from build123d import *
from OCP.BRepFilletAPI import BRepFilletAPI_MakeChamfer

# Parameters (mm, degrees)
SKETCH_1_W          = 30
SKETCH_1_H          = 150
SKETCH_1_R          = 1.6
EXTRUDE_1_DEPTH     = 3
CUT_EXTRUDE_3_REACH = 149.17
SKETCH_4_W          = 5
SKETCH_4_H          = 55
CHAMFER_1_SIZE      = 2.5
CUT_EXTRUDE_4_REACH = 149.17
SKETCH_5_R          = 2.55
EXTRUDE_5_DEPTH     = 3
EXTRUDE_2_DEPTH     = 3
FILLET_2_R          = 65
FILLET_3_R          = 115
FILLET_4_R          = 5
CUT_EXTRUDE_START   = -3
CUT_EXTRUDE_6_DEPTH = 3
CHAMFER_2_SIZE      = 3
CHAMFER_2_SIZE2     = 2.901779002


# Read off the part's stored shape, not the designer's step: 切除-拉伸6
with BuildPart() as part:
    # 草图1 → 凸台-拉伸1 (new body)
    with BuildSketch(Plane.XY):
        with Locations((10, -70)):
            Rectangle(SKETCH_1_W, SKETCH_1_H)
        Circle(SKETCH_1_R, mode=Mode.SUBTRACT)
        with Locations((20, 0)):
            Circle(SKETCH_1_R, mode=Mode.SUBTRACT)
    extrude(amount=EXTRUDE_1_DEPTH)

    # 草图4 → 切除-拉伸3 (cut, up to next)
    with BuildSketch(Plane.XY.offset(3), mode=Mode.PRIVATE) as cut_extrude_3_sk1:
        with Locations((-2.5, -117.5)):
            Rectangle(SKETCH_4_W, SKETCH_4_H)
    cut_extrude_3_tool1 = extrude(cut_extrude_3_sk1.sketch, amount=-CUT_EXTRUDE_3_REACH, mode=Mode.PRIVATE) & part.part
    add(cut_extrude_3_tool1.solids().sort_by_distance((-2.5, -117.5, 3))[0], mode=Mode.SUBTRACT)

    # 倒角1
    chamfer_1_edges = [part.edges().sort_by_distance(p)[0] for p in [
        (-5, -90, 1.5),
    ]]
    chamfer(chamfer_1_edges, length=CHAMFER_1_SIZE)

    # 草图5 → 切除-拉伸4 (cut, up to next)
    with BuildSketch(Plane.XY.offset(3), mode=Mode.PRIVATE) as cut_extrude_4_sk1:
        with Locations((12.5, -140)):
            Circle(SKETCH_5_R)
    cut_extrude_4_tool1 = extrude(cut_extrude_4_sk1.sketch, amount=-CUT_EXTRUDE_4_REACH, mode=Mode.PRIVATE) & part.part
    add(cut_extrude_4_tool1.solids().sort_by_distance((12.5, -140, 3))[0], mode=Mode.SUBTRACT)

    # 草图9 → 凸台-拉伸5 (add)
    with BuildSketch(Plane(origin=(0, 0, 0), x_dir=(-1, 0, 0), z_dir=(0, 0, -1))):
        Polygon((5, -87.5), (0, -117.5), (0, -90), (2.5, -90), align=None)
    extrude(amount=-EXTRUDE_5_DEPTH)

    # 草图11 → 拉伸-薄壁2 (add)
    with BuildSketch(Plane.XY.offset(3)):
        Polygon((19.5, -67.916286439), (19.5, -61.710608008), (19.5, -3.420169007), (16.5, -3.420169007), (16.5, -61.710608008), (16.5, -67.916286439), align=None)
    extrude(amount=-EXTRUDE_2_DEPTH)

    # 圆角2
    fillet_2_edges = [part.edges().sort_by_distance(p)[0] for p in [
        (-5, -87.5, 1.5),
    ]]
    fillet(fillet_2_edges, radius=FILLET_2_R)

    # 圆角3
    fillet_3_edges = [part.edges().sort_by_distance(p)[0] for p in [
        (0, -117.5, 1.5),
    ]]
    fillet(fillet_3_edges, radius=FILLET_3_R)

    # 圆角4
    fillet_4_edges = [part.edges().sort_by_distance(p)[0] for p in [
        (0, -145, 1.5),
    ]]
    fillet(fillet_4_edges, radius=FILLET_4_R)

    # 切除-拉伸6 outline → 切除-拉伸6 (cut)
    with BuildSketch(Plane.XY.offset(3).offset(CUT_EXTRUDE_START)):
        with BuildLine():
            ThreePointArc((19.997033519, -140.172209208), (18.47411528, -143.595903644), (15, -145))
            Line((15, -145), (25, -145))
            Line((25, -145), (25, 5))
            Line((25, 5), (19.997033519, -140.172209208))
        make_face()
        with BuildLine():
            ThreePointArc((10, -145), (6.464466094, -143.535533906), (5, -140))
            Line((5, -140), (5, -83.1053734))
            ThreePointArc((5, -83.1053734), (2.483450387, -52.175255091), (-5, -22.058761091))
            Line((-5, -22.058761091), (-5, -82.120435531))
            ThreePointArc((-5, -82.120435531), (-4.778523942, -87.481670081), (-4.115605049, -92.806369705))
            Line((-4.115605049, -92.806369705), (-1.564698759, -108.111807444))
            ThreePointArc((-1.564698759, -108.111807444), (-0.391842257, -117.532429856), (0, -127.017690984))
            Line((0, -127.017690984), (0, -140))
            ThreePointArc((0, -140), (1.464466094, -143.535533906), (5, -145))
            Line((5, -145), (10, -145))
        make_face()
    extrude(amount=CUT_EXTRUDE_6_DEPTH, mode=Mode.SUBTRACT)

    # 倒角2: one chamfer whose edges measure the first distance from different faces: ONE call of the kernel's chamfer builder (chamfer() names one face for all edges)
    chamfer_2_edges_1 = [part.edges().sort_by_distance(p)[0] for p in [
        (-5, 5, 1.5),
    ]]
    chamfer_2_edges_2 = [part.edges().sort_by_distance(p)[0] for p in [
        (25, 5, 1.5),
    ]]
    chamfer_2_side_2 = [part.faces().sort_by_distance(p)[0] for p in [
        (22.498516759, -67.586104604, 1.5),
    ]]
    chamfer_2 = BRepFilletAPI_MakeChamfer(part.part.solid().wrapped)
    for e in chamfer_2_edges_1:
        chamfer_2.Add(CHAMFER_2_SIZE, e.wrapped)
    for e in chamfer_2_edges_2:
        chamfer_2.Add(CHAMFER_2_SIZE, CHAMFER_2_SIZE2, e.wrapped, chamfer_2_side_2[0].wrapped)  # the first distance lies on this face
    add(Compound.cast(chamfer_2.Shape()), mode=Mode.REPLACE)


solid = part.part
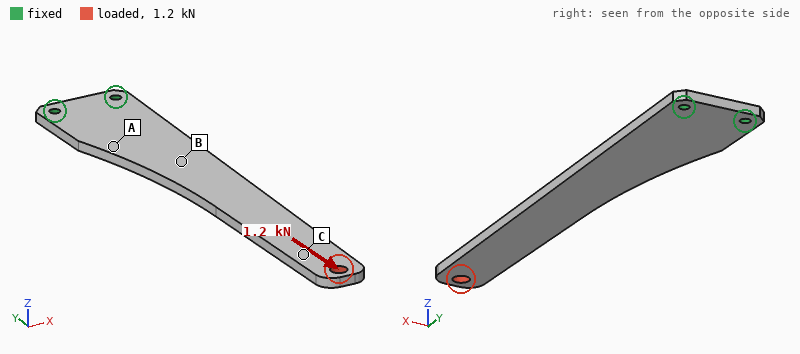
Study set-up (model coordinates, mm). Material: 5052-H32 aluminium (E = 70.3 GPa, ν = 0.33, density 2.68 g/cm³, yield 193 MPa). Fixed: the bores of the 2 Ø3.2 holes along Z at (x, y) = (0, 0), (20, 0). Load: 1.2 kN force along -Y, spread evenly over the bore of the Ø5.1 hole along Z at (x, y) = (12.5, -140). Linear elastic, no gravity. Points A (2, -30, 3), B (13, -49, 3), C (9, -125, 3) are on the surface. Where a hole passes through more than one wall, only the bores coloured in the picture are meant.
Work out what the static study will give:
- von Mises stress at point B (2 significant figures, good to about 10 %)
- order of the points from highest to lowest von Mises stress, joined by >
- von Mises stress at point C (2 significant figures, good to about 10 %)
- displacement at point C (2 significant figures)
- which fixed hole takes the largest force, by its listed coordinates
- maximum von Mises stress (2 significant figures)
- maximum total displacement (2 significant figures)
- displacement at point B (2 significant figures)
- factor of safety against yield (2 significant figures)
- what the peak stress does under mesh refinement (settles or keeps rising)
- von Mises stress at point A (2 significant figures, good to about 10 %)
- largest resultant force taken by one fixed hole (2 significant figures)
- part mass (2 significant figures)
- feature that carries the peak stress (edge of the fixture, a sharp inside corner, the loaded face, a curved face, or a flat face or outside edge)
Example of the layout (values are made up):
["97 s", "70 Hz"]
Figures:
["19 MPa", "C > B > A", "27 MPa", "39 µm", "(20, 0)", "86 MPa", "49 µm", "15 µm", "2.2", "settles", "11 MPa", "750 N", "24 g", "the loaded face"]
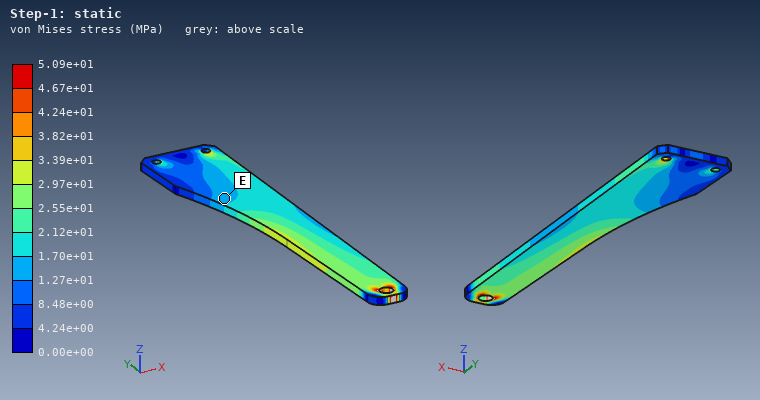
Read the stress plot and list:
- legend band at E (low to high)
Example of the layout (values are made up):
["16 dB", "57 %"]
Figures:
["1.27e+01 to 1.70e+01 MPa"]
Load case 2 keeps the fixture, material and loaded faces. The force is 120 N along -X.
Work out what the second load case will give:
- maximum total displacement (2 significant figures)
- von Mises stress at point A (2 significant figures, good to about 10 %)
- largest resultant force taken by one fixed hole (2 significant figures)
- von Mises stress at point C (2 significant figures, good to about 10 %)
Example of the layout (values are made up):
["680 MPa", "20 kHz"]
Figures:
["0.58 mm", "26 MPa", "790 N", "8.2 MPa"]
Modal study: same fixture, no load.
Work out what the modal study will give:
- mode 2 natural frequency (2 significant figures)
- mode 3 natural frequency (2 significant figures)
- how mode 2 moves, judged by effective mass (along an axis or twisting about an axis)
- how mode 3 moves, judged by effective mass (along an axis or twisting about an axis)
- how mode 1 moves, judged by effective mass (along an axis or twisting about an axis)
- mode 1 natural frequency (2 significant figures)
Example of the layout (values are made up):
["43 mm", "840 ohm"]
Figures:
["810 Hz", "1200 Hz", "along Z", "along X", "along Z", "150 Hz"]
